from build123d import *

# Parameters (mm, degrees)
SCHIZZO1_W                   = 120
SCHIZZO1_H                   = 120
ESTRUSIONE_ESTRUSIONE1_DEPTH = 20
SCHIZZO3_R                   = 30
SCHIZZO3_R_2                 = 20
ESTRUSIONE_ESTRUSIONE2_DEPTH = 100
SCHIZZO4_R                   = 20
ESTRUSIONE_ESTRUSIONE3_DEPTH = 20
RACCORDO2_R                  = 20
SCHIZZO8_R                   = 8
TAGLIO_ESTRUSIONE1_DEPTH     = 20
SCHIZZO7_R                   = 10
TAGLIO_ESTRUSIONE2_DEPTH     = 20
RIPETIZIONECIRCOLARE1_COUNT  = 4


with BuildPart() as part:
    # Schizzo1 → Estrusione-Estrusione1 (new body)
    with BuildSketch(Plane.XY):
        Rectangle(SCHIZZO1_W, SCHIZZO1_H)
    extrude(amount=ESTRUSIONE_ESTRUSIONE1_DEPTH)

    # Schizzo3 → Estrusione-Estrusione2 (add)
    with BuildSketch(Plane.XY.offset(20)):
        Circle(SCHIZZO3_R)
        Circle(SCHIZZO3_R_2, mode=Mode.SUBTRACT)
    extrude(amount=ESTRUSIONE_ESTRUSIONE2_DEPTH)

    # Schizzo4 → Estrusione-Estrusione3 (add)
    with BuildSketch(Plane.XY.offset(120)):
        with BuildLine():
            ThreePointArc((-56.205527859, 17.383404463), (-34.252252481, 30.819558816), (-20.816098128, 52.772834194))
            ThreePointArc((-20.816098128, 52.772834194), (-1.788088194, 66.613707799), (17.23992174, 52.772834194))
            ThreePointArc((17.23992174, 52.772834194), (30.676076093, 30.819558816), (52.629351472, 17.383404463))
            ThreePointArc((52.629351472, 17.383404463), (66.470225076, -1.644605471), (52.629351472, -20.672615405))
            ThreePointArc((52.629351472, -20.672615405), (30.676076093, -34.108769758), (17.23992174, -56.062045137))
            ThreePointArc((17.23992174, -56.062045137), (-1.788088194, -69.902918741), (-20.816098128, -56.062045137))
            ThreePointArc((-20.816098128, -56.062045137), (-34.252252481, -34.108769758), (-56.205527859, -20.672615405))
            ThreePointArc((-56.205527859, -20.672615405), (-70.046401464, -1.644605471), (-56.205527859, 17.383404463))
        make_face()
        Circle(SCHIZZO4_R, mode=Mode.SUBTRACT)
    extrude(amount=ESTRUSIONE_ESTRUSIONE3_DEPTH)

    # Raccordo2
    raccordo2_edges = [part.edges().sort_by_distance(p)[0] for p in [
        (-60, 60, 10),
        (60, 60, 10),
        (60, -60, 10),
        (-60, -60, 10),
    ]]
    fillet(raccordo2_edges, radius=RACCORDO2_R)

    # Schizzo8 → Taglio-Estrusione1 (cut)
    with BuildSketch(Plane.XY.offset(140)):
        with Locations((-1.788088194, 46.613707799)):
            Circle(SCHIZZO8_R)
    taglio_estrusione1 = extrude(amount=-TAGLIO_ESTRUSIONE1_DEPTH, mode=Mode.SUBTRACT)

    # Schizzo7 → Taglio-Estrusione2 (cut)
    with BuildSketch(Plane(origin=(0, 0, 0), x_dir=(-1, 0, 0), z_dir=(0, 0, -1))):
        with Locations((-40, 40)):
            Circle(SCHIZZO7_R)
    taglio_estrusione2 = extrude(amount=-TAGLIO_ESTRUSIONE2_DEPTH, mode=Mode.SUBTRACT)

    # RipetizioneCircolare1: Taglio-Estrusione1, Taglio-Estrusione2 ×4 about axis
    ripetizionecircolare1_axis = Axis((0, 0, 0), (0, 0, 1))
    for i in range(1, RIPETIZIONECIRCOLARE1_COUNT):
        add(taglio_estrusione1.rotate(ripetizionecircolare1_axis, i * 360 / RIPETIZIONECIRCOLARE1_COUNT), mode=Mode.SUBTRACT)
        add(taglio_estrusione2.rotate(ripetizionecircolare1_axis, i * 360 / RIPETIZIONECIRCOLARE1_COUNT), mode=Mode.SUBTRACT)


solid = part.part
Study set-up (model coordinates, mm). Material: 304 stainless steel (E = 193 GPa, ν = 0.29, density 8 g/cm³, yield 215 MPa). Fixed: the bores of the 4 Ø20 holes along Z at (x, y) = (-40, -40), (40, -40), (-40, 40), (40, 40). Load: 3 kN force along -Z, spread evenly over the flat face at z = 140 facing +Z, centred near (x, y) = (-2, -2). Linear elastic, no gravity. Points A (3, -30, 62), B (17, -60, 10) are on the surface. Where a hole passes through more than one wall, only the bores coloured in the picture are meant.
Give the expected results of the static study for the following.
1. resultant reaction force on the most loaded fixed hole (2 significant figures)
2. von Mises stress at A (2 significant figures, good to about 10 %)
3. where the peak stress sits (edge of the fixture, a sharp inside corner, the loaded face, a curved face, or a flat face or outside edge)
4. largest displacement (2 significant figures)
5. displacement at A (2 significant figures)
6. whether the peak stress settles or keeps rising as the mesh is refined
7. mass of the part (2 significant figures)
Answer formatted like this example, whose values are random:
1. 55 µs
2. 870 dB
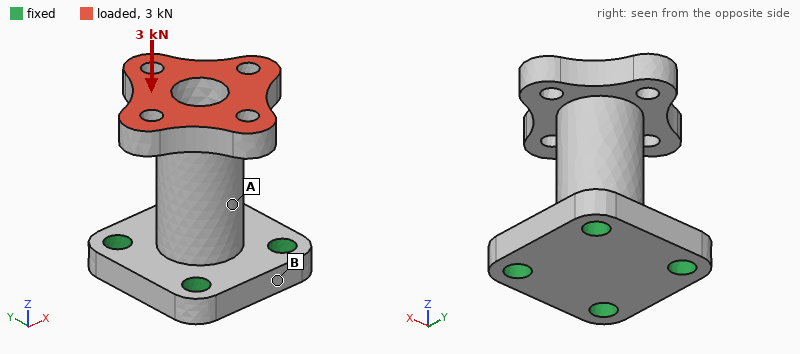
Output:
1. 860 N
2. 2.2 MPa
3. edge of the fixture
4. 4.7 µm
5. 1.1 µm
6. keeps rising
7. 4.6 kg
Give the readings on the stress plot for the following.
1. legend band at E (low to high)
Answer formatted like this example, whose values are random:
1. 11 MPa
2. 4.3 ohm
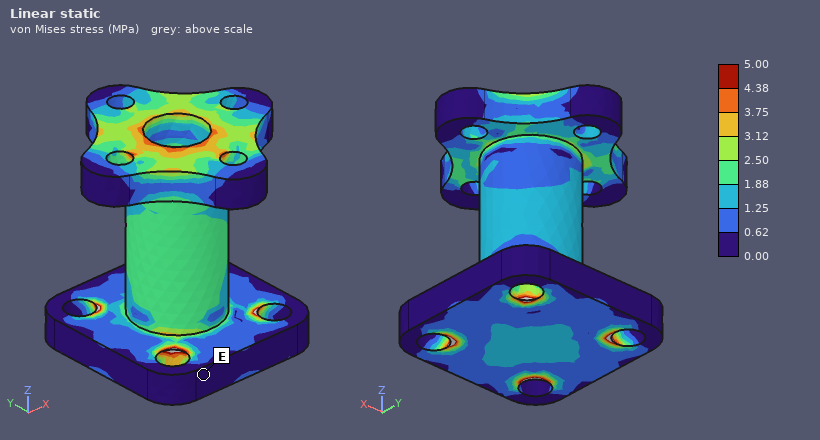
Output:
1. 0.00 to 0.62 MPa
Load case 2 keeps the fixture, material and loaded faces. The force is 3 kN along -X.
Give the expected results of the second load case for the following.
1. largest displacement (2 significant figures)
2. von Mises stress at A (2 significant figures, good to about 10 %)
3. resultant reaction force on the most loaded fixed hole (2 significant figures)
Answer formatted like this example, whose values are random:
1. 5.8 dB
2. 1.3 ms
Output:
1. 42 µm
2. 6.0 MPa
3. 3.0 kN
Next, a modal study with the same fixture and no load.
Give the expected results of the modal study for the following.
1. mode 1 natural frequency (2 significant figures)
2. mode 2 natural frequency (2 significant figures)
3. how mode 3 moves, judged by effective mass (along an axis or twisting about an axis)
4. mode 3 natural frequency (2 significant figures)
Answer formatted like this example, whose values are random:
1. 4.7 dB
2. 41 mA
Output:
1. 1300 Hz
2. 1300 Hz
3. twisting about Z
4. 2500 Hz
